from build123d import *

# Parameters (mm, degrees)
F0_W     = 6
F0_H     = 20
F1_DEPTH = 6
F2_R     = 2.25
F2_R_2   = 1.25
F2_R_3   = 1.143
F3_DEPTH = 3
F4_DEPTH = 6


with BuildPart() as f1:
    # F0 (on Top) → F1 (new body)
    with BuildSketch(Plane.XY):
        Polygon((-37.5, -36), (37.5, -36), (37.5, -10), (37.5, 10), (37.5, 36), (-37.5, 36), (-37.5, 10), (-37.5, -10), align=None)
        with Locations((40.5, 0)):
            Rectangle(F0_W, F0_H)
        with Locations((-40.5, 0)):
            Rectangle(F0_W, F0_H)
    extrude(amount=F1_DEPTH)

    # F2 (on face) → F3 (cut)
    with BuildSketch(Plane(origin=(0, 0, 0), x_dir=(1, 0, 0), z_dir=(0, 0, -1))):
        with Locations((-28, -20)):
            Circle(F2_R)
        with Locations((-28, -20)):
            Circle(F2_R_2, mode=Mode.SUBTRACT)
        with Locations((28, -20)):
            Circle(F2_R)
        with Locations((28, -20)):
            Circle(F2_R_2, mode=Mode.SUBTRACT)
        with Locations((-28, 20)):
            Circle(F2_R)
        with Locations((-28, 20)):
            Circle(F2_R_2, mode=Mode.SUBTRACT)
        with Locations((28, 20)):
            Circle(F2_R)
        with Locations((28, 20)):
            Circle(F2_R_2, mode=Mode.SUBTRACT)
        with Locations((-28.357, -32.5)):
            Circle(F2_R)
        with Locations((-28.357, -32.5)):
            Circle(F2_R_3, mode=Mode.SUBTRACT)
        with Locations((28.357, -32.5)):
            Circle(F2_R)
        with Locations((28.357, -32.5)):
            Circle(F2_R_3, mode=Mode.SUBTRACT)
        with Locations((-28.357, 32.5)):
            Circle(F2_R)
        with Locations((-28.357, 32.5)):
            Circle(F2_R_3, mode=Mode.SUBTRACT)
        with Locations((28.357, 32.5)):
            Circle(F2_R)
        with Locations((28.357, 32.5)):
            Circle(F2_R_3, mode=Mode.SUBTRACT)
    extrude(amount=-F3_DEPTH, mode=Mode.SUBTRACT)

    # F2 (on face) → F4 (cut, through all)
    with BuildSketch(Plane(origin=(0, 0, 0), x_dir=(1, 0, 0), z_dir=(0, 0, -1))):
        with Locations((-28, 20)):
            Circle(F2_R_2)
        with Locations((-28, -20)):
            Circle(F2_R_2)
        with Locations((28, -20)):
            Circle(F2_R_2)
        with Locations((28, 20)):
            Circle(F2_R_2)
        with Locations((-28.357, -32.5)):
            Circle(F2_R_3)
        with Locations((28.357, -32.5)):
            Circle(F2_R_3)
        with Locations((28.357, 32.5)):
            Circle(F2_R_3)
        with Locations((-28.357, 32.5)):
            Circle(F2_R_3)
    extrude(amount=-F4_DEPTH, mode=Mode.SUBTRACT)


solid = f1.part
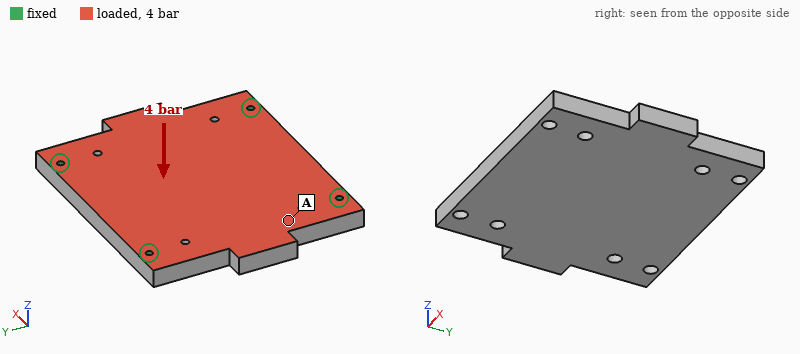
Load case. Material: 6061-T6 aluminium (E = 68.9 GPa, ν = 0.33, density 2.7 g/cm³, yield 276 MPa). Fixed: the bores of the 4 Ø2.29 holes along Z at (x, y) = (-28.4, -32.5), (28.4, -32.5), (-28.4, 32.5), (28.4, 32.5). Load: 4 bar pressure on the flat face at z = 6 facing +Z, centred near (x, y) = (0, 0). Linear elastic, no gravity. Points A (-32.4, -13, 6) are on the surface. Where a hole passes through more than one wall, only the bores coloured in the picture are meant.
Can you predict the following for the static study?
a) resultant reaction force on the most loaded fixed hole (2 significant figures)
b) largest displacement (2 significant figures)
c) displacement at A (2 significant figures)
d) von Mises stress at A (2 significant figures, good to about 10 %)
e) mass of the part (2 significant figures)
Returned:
810 N
58 µm
37 µm
18 MPa
90 g
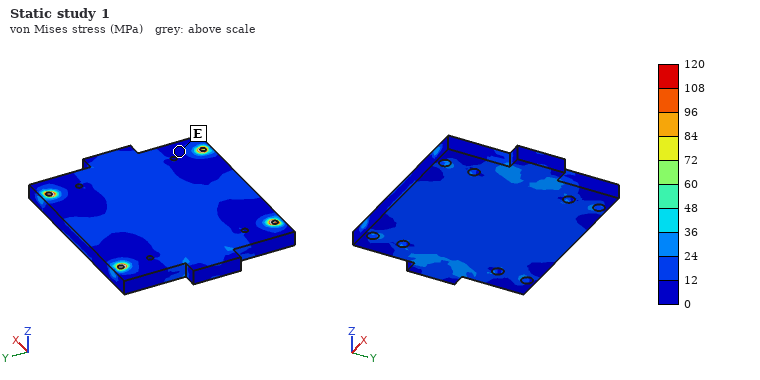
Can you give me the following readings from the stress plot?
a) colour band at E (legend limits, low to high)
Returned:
0 to 12 MPa
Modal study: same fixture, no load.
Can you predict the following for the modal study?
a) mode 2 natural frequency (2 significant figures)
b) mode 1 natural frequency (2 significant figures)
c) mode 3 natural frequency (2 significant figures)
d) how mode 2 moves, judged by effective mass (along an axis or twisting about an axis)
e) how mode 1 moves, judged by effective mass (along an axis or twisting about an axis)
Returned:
5100 Hz
3800 Hz
5900 Hz
twisting about Y
along Z
